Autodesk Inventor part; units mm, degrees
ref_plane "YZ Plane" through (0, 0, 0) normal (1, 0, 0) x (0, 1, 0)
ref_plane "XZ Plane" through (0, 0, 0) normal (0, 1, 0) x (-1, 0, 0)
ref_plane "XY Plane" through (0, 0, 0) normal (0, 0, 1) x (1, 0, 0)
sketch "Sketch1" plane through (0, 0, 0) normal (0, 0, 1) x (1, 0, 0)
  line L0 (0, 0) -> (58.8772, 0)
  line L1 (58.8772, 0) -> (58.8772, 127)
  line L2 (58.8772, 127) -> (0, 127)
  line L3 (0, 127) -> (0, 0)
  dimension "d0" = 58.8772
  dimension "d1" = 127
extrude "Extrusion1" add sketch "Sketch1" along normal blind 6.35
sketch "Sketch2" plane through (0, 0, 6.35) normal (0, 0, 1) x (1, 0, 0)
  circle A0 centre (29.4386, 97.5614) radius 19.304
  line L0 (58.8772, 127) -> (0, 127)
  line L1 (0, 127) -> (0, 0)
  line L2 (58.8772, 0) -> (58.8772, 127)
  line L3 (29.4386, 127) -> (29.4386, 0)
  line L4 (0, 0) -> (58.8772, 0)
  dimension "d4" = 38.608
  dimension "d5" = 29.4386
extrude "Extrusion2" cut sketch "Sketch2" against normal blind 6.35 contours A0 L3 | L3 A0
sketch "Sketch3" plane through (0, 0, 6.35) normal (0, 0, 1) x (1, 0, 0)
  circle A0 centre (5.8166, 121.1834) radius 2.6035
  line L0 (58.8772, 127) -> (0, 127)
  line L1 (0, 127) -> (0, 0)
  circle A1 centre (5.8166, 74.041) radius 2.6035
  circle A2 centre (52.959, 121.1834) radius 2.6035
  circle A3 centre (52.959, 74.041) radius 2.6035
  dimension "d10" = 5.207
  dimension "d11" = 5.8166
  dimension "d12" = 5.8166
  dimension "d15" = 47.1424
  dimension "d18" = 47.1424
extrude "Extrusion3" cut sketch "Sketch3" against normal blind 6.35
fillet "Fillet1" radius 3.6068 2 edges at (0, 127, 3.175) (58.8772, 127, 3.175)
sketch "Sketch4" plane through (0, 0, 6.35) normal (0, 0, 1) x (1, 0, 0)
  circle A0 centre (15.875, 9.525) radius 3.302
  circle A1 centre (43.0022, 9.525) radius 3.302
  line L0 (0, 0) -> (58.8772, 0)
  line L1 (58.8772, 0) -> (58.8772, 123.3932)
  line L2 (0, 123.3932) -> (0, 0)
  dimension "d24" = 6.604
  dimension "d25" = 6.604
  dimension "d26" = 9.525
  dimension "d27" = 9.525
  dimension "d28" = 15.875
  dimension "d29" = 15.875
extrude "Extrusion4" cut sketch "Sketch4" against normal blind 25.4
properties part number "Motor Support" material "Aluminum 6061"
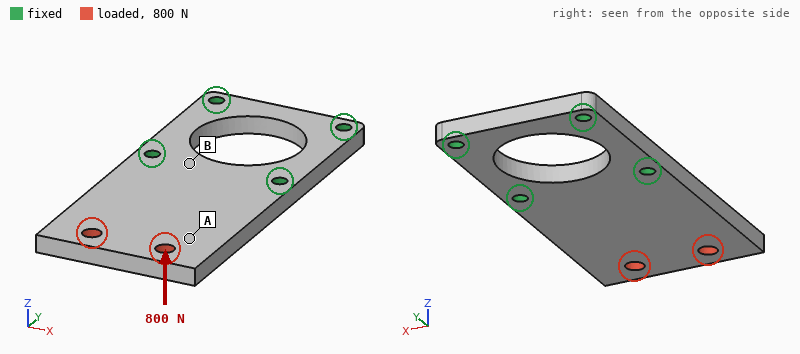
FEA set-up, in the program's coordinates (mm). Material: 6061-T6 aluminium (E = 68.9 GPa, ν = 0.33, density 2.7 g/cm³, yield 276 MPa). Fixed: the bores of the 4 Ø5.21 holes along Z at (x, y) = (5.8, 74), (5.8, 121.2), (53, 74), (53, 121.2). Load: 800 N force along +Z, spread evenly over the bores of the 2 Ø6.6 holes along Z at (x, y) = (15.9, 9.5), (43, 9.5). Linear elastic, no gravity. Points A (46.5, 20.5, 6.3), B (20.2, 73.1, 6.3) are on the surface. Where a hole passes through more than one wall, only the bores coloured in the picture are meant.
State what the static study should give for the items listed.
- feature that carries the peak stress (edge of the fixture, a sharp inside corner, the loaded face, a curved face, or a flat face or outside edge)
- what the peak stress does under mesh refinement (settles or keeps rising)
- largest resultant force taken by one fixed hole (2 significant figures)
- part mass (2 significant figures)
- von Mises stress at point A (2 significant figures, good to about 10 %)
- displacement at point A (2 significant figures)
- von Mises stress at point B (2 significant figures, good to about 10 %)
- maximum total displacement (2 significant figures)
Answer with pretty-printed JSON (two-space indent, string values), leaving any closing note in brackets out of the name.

{
  "feature that carries the peak stress": "edge of the fixture",
  "what the peak stress does under mesh refinement": "keeps rising",
  "largest resultant force taken by one fixed hole": "480 N",
  "part mass": "110 g",
  "von Mises stress at point A": "27 MPa",
  "displacement at point A": "0.72 mm",
  "von Mises stress at point B": "74 MPa",
  "maximum total displacement": "1.2 mm"
}
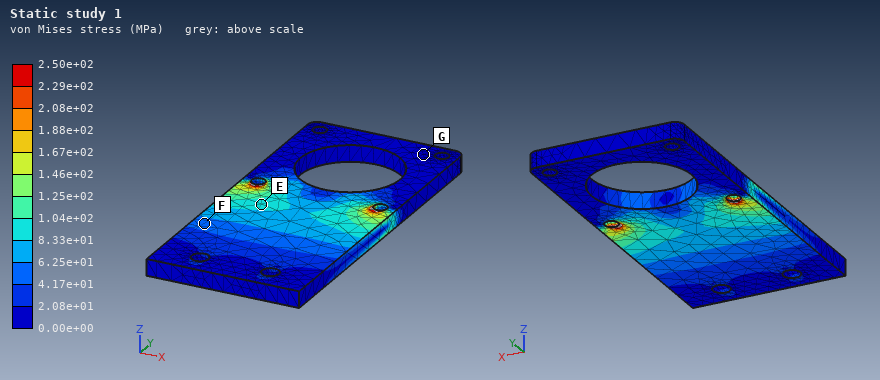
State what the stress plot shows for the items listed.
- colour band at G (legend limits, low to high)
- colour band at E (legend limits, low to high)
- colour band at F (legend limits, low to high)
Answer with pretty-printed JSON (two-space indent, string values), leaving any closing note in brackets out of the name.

{
  "colour band at G": "0.00e+00 to 2.08e+01 MPa",
  "colour band at E": "8.33e+01 to 1.04e+02 MPa",
  "colour band at F": "4.17e+01 to 6.25e+01 MPa"
}
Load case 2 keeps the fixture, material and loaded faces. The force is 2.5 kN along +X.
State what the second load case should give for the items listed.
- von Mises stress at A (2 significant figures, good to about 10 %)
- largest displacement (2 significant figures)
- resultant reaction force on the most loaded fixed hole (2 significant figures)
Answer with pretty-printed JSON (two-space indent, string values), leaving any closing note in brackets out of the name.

{
  "von Mises stress at A": "13 MPa",
  "largest displacement": "63 µm",
  "resultant reaction force on the most loaded fixed hole": "3.5 kN"
}
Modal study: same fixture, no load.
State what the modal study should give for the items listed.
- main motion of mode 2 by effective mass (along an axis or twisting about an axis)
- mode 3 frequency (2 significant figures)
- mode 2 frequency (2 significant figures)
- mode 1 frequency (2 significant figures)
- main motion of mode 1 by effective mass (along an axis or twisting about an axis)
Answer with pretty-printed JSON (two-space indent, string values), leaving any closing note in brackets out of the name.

{
  "main motion of mode 2 by effective mass": "twisting about Y",
  "mode 3 frequency": "5500 Hz",
  "mode 2 frequency": "2700 Hz",
  "mode 1 frequency": "890 Hz",
  "main motion of mode 1 by effective mass": "along Z"
}
